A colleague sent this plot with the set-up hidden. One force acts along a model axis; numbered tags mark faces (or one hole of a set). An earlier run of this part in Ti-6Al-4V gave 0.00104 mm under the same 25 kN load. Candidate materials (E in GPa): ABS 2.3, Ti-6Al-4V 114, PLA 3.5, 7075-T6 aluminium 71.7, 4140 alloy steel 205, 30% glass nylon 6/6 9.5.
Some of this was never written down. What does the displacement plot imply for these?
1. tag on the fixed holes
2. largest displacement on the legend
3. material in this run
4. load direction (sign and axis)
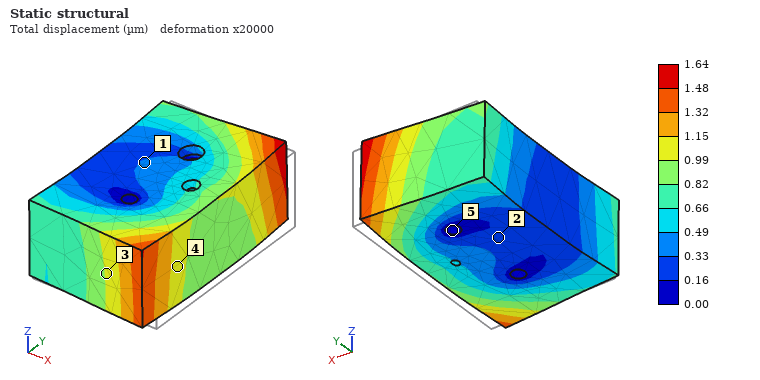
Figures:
5
1.64 µm
7075-T6 aluminium
-X
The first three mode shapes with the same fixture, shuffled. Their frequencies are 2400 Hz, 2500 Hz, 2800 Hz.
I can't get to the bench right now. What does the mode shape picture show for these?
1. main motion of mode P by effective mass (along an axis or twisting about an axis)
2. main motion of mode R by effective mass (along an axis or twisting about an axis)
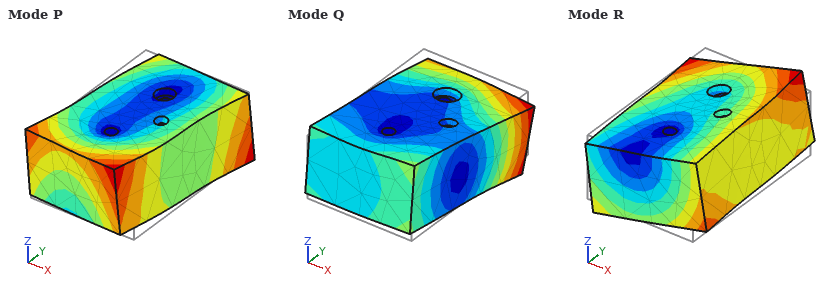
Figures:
twisting about Z
twisting about Y
